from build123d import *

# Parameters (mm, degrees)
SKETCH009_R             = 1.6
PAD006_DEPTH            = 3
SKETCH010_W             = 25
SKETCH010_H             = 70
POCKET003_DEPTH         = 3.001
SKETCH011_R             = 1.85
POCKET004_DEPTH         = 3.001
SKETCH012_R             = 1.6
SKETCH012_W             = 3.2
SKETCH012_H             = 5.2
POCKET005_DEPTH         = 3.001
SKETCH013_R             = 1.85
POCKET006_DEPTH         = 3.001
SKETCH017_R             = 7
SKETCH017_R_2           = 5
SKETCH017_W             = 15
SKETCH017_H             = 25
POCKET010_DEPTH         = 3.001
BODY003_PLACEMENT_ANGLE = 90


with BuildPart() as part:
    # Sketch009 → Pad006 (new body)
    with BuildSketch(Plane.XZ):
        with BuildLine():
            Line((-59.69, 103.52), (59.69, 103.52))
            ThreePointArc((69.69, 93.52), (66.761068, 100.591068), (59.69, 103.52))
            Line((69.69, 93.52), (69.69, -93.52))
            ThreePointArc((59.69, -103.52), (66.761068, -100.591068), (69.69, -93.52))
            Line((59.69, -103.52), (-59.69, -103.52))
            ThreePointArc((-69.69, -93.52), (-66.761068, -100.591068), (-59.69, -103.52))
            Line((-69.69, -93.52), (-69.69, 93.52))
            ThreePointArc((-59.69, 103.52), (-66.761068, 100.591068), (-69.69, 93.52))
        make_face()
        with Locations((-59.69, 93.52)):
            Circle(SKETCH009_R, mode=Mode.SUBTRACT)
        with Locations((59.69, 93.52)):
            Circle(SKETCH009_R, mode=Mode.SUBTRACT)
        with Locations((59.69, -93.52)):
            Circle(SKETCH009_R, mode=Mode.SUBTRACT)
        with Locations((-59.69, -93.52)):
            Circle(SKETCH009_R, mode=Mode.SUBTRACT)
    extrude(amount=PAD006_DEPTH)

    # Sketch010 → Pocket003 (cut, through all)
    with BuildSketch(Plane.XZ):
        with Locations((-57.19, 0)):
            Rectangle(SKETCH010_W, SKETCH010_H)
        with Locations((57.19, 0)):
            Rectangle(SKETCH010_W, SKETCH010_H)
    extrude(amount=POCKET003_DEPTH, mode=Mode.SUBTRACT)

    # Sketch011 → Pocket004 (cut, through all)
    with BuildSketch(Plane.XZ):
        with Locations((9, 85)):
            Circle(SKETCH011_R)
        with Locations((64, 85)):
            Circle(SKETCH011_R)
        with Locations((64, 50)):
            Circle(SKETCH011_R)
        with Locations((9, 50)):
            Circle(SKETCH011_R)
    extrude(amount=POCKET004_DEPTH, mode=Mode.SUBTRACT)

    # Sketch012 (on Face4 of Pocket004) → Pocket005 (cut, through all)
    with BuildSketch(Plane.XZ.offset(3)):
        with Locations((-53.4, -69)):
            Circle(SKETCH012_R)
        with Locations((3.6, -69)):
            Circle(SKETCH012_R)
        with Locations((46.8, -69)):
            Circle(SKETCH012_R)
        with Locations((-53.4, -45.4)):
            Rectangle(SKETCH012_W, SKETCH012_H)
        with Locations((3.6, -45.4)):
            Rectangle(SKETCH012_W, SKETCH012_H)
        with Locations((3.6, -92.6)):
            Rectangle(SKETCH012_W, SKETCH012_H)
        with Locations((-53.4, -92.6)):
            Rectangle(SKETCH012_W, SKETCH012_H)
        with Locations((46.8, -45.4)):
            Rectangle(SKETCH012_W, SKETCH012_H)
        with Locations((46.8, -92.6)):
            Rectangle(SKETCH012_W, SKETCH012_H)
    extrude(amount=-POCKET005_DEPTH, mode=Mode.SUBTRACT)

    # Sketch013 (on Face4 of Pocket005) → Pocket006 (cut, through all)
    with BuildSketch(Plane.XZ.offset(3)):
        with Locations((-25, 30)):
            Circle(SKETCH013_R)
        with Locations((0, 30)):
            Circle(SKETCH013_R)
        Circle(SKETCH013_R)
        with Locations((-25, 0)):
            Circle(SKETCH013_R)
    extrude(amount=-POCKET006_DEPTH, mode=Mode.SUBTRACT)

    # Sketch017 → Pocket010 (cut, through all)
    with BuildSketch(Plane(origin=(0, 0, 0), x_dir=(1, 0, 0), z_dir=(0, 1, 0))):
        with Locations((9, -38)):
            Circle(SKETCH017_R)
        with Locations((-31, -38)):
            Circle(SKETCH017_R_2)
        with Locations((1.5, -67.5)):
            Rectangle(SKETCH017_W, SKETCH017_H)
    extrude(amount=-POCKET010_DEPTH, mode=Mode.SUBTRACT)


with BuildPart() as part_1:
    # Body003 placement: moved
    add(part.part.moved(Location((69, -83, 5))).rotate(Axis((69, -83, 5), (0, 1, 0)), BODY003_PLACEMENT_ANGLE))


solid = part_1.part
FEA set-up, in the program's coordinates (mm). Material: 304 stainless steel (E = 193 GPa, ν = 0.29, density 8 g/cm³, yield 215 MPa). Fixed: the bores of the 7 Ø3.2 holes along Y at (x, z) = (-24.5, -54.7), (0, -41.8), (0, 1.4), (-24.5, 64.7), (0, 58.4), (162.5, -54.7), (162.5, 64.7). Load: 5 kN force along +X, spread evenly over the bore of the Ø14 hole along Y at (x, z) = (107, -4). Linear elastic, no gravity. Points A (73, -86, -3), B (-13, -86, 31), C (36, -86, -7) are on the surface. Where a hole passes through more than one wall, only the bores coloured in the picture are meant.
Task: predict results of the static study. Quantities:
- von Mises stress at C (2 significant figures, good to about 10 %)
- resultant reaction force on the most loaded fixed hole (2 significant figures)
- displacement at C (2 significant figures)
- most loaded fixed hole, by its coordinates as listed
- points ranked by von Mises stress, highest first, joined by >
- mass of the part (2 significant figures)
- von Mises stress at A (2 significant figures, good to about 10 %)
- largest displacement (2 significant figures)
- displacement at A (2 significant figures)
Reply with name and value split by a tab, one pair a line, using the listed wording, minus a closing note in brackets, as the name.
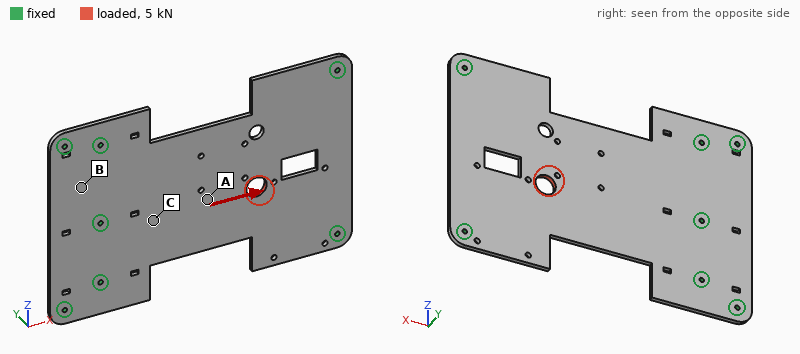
von Mises stress at C	10 MPa
resultant reaction force on the most loaded fixed hole	1.4 kN
displacement at C	2.7 µm
most loaded fixed hole, by its coordinates as listed	(162.5, -54.7)
points ranked by von Mises stress, highest first, joined by >	A > C > B
mass of the part	590 g
von Mises stress at A	20 MPa
largest displacement	12 µm
displacement at A	5.2 µm
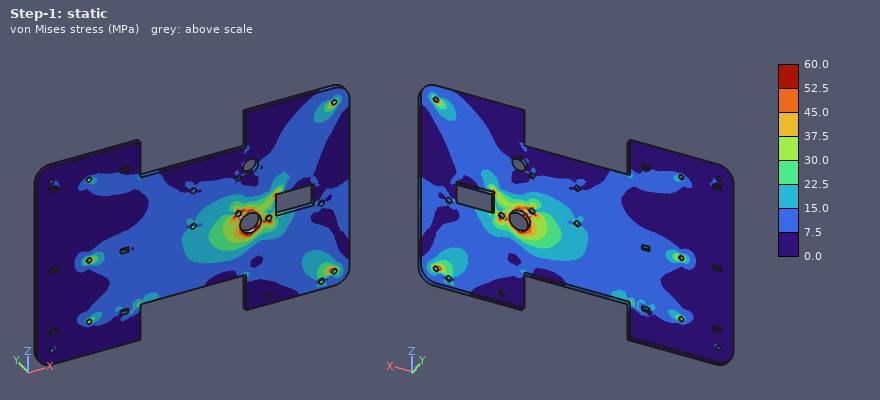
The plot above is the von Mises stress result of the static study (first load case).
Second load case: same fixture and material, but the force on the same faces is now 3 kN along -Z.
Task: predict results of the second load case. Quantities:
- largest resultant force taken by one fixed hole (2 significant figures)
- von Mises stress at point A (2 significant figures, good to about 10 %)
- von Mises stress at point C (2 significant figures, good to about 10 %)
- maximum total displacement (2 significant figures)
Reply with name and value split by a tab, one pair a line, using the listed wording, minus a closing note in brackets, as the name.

largest resultant force taken by one fixed hole	1.2 kN
von Mises stress at point A	6.0 MPa
von Mises stress at point C	5.6 MPa
maximum total displacement	11 µm
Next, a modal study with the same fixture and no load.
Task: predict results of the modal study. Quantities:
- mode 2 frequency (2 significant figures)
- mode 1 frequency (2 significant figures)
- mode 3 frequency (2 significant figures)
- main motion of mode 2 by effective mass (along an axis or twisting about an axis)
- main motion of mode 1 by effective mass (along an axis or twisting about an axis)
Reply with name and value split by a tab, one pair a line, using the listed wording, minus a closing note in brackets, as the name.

mode 2 frequency	860 Hz
mode 1 frequency	480 Hz
mode 3 frequency	1000 Hz
main motion of mode 2 by effective mass	twisting about X
main motion of mode 1 by effective mass	along Y
